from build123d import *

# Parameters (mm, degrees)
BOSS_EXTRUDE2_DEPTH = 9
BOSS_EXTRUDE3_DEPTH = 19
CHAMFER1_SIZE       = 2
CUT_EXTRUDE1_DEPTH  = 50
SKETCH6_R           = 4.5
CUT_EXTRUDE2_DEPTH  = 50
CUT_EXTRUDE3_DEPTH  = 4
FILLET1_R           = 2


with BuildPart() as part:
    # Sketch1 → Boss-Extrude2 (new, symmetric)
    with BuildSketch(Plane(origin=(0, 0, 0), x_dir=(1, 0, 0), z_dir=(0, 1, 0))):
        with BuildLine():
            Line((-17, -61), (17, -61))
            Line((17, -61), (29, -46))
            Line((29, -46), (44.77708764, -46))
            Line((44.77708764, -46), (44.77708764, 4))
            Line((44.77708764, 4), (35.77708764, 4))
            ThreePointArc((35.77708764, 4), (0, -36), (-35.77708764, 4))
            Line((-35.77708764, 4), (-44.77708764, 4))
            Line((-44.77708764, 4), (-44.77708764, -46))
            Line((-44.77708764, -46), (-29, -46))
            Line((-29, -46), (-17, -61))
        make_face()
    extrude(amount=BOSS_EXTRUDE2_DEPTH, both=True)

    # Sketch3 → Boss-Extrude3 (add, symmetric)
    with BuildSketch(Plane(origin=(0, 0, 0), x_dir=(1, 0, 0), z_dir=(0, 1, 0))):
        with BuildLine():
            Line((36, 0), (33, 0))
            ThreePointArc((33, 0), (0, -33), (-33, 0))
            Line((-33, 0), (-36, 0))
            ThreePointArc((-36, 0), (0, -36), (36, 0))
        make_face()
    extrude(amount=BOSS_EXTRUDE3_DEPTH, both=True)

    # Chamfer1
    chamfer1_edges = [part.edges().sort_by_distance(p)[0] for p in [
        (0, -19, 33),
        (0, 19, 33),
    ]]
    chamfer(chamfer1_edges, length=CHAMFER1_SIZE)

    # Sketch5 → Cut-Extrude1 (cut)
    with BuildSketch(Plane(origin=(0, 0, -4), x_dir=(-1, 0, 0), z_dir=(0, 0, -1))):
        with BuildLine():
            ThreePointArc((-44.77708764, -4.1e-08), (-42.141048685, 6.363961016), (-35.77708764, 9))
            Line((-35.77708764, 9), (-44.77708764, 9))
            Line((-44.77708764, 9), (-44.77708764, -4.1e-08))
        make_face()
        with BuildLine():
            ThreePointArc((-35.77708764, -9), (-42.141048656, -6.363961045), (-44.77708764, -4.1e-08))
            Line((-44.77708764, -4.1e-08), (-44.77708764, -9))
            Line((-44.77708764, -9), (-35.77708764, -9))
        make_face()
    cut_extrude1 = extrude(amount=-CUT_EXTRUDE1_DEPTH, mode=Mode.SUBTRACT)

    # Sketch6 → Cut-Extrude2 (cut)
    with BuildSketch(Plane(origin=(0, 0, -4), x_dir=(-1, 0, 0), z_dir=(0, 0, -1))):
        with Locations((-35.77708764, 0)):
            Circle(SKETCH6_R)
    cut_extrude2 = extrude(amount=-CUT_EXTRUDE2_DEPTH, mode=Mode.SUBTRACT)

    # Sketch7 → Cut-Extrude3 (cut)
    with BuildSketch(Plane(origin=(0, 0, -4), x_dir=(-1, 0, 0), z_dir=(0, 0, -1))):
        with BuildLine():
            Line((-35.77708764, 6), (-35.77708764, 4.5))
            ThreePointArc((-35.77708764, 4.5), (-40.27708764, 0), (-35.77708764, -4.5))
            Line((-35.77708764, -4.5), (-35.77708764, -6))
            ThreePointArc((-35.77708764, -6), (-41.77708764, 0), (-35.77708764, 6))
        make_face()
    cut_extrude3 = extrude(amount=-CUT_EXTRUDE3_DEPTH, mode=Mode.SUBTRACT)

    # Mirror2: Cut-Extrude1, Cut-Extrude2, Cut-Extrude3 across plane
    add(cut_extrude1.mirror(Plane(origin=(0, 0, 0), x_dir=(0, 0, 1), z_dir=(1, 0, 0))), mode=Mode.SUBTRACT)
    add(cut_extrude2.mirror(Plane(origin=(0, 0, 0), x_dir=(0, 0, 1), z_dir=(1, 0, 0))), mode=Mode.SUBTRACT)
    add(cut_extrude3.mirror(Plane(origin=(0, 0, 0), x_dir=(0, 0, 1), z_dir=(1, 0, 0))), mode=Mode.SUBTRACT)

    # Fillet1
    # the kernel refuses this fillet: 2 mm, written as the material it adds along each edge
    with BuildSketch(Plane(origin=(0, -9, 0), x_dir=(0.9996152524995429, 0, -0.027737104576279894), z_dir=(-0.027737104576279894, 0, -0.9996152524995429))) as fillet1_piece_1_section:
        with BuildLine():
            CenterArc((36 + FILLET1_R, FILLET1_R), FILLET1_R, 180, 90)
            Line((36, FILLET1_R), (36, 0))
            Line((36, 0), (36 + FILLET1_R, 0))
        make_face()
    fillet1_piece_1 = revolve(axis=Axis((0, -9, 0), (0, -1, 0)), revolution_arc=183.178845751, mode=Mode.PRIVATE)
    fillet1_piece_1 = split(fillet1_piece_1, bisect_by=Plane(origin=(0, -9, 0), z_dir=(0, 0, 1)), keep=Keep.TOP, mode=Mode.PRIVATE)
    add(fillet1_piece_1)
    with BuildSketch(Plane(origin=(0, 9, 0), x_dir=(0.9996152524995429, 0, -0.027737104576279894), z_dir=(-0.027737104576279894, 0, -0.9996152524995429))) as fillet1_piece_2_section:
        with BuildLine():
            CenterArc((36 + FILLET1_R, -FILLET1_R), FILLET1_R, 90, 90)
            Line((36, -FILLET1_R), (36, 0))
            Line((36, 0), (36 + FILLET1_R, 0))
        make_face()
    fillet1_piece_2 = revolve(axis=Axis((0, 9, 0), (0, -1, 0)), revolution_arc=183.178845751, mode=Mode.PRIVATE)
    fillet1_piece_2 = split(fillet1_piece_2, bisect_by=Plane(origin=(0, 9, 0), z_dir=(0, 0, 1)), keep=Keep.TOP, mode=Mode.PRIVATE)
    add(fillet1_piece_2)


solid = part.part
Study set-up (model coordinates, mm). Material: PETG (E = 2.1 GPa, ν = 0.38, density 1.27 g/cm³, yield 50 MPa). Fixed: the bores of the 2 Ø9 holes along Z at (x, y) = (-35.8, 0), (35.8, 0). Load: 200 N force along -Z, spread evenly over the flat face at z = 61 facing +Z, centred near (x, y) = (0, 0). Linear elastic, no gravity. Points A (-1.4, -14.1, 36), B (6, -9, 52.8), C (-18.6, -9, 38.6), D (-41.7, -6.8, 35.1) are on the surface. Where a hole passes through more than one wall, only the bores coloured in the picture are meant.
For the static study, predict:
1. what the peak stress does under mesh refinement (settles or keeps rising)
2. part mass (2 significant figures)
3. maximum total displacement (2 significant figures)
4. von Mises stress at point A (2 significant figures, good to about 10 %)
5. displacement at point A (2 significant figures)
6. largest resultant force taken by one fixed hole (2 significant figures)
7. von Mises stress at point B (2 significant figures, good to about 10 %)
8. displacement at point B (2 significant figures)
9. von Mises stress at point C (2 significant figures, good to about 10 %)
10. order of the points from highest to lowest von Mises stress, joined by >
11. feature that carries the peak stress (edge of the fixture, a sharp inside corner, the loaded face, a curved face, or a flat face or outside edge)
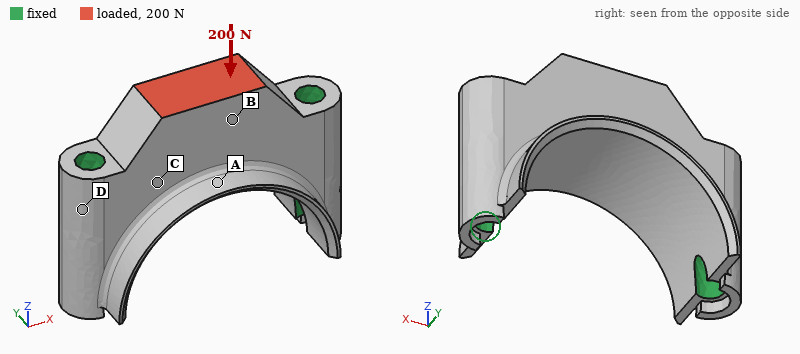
keeps rising
68 g
9.8 µm
0.14 MPa
7.6 µm
120 N
0.28 MPa
8.6 µm
0.37 MPa
C > B > A > D
edge of the fixture
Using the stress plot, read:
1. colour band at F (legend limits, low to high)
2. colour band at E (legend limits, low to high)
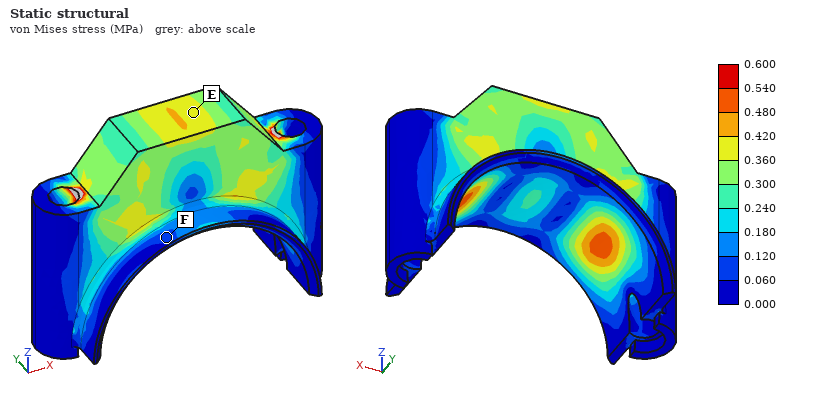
0.060 to 0.120 MPa
0.360 to 0.420 MPa
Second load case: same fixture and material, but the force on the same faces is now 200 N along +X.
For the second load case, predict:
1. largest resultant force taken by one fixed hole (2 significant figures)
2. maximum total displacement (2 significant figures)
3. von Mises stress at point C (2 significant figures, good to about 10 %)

130 N
9.8 µm
0.19 MPa
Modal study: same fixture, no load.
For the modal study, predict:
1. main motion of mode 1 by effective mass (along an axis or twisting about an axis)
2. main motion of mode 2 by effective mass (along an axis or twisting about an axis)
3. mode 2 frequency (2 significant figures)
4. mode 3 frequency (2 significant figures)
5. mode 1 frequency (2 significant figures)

along Y
along Z
4700 Hz
5100 Hz
2600 Hz
